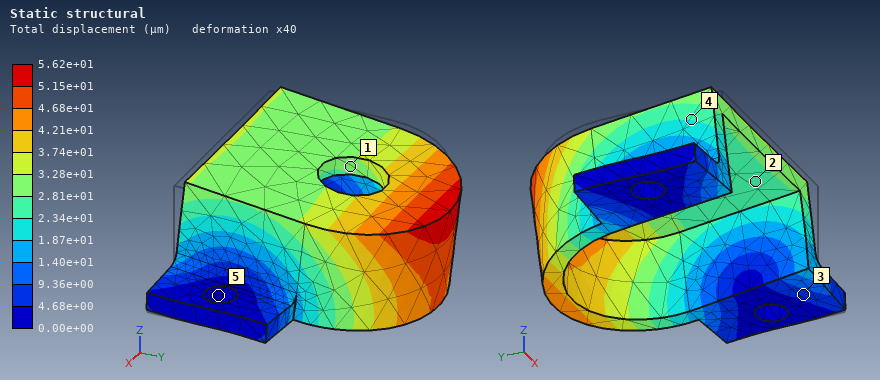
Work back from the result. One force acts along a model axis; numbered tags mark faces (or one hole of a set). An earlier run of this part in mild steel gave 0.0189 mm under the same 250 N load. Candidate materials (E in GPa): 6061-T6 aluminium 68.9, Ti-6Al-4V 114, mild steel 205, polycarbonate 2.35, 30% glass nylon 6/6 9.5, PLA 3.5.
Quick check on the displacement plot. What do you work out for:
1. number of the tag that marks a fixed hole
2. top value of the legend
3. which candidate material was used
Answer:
5
5.62e+01 µm
6061-T6 aluminium
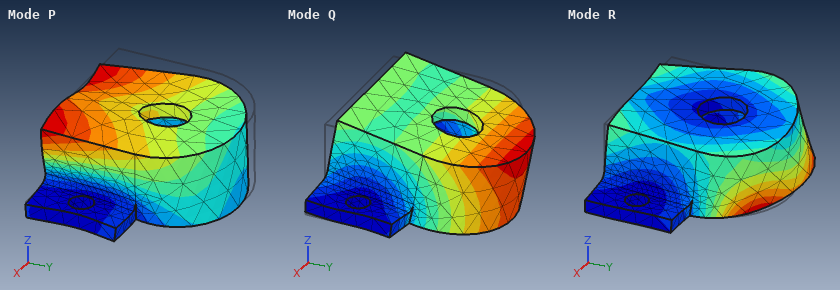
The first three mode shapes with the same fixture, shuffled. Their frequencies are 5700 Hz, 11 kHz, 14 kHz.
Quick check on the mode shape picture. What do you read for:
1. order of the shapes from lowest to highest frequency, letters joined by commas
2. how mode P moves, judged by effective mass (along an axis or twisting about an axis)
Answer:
Q, P, R
along X
